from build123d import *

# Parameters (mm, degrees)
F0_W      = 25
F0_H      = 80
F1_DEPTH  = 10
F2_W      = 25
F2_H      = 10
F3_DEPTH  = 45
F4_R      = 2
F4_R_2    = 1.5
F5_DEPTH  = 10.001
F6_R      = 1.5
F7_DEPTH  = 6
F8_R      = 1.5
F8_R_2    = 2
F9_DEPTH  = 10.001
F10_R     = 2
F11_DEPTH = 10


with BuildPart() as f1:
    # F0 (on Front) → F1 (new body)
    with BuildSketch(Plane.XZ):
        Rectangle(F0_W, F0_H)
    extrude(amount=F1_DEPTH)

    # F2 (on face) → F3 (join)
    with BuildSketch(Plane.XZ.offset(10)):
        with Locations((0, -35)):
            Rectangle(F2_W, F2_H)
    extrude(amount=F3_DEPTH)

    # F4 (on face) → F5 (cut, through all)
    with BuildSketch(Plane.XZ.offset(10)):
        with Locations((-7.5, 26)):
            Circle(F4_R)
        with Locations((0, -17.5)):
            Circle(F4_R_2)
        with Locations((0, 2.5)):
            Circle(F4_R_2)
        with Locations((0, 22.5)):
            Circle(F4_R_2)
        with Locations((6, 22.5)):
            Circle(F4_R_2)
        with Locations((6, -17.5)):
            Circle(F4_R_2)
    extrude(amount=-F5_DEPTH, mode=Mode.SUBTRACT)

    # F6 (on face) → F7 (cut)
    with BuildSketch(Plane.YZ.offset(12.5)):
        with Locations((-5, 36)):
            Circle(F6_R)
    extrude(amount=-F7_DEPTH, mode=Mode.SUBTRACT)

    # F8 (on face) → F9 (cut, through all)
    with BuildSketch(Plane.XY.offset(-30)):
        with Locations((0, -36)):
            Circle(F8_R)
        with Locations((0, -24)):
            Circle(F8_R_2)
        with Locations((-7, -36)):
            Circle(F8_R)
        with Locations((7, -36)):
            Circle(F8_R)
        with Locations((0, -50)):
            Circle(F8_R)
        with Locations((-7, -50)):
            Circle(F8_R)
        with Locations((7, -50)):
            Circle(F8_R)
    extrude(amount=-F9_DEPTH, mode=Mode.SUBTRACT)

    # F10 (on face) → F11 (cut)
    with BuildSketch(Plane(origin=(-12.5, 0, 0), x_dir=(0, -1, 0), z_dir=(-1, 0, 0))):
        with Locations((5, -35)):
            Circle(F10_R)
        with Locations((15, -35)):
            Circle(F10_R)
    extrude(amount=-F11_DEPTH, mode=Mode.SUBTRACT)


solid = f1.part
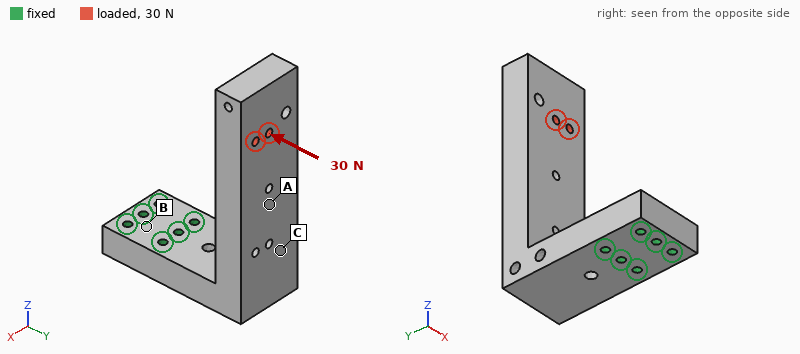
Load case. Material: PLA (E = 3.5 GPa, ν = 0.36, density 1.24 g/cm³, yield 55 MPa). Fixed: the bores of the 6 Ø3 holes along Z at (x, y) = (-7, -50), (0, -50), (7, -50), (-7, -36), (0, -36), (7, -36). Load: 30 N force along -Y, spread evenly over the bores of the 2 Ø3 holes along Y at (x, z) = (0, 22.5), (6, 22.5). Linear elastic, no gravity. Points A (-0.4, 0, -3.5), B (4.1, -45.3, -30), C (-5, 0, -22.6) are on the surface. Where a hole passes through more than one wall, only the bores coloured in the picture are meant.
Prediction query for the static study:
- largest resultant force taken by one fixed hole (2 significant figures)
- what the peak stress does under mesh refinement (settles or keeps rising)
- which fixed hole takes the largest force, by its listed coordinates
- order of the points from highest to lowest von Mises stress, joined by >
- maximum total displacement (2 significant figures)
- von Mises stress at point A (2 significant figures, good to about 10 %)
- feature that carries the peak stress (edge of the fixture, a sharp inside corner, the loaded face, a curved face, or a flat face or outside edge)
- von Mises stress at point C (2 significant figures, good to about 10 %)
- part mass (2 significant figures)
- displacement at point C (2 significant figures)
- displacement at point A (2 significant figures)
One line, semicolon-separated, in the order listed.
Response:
20 N; keeps rising; (0, -36); C > A > B; 0.94 mm; 1.7 MPa; a sharp inside corner; 3.3 MPa; 37 g; 0.19 mm; 0.37 mm
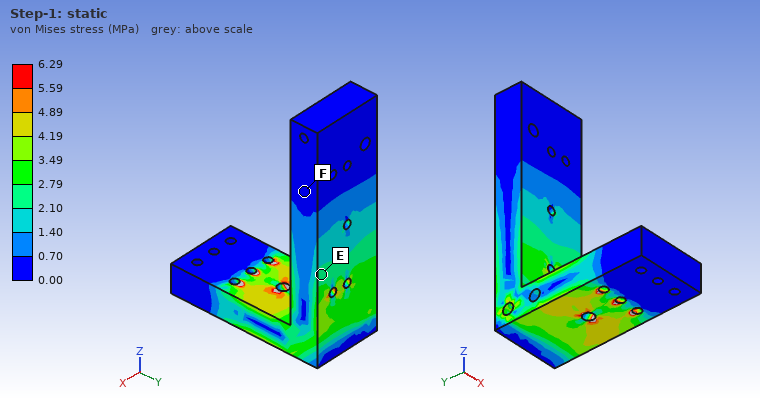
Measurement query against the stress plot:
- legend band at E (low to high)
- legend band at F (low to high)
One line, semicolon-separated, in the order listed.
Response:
2.10 to 2.79 MPa; 0.00 to 0.70 MPa
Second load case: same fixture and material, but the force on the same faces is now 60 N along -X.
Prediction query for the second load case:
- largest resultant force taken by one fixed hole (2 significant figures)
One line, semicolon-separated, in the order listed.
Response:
180 N
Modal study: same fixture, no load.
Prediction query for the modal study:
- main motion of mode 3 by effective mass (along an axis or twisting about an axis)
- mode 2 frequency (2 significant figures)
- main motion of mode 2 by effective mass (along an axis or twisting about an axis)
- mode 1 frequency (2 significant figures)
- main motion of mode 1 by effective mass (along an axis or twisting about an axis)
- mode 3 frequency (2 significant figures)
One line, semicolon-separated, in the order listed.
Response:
along Z; 400 Hz; along X; 290 Hz; along Y; 1100 Hz
